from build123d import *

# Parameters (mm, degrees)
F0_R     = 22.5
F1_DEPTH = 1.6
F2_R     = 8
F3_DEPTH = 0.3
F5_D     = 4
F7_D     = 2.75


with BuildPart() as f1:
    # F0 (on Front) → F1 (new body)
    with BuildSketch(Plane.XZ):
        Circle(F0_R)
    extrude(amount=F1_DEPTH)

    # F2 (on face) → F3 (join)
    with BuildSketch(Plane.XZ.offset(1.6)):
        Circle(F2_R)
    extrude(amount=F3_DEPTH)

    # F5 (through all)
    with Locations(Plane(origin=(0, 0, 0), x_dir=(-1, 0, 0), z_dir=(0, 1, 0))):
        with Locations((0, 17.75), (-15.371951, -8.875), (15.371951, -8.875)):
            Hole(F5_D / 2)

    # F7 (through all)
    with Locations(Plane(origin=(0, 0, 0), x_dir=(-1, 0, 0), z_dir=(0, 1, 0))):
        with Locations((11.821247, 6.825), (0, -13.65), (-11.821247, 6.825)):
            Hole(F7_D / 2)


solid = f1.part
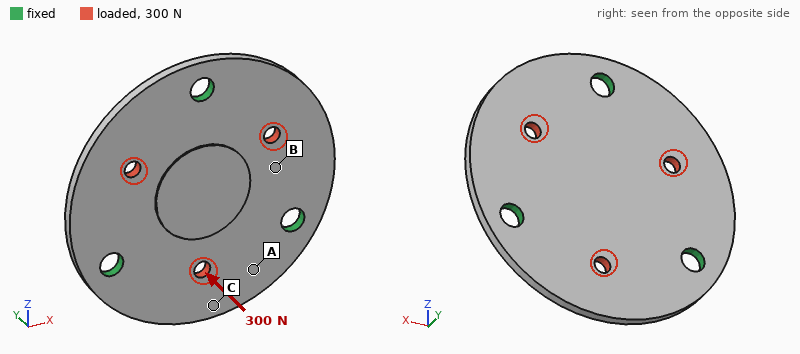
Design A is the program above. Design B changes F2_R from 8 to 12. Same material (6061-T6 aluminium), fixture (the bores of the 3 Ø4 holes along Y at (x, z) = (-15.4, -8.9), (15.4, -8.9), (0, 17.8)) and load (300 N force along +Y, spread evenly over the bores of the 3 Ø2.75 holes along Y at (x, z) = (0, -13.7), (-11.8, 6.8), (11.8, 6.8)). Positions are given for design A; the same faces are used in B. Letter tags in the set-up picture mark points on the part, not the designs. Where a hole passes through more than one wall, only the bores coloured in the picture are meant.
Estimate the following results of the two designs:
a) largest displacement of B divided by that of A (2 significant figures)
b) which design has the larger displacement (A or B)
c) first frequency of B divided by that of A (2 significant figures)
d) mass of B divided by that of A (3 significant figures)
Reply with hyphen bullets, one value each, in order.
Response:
- 0.91
- A
- 1.0
- 1.03
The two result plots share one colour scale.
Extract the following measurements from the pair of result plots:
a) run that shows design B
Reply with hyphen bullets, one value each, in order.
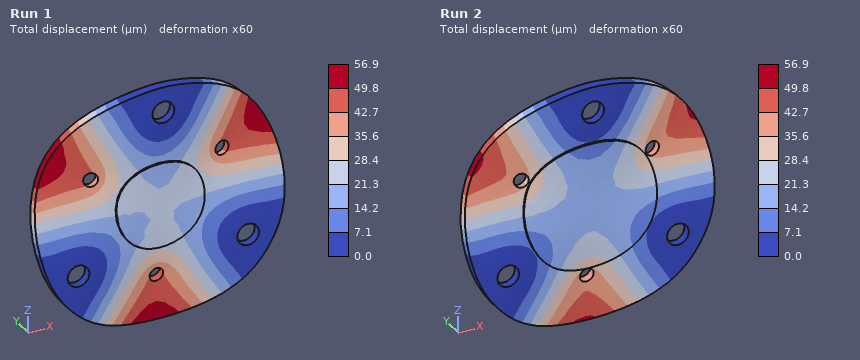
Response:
- Run 2
